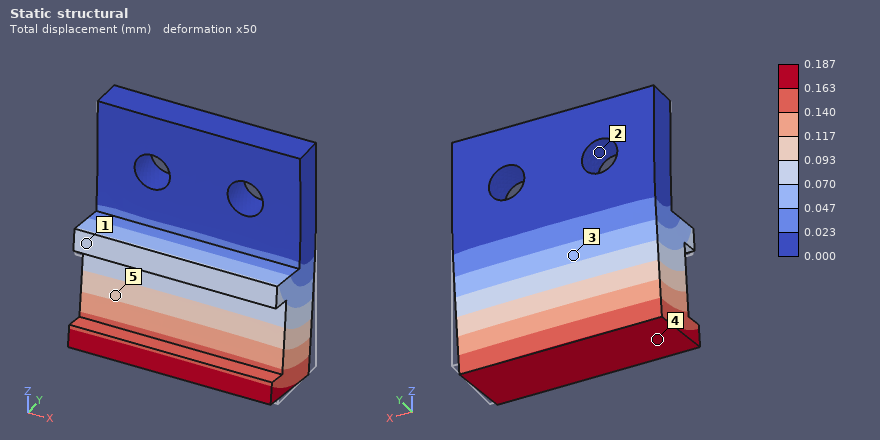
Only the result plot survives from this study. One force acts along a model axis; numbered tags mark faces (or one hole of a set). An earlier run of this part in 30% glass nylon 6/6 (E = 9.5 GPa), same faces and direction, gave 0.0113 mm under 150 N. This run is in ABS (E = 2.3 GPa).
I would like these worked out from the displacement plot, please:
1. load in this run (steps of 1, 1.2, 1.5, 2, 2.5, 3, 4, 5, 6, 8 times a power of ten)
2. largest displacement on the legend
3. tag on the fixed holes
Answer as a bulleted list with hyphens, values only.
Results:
- 600 N
- 0.187 mm
- 2
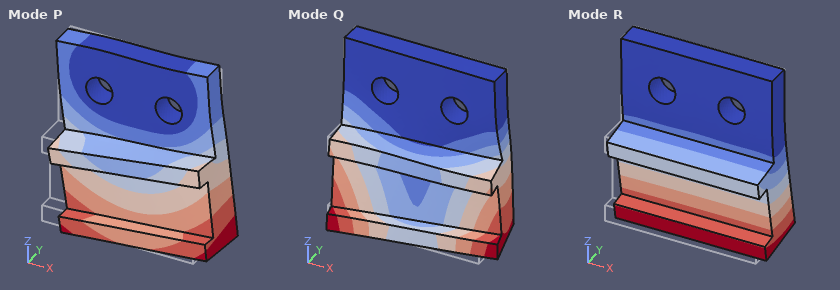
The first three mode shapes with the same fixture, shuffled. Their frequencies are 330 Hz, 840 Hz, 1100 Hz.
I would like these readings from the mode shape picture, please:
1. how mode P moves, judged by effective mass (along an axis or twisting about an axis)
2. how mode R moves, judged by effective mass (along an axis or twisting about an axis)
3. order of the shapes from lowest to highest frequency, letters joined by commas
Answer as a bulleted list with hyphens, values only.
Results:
- along X
- along Y
- R, Q, P
